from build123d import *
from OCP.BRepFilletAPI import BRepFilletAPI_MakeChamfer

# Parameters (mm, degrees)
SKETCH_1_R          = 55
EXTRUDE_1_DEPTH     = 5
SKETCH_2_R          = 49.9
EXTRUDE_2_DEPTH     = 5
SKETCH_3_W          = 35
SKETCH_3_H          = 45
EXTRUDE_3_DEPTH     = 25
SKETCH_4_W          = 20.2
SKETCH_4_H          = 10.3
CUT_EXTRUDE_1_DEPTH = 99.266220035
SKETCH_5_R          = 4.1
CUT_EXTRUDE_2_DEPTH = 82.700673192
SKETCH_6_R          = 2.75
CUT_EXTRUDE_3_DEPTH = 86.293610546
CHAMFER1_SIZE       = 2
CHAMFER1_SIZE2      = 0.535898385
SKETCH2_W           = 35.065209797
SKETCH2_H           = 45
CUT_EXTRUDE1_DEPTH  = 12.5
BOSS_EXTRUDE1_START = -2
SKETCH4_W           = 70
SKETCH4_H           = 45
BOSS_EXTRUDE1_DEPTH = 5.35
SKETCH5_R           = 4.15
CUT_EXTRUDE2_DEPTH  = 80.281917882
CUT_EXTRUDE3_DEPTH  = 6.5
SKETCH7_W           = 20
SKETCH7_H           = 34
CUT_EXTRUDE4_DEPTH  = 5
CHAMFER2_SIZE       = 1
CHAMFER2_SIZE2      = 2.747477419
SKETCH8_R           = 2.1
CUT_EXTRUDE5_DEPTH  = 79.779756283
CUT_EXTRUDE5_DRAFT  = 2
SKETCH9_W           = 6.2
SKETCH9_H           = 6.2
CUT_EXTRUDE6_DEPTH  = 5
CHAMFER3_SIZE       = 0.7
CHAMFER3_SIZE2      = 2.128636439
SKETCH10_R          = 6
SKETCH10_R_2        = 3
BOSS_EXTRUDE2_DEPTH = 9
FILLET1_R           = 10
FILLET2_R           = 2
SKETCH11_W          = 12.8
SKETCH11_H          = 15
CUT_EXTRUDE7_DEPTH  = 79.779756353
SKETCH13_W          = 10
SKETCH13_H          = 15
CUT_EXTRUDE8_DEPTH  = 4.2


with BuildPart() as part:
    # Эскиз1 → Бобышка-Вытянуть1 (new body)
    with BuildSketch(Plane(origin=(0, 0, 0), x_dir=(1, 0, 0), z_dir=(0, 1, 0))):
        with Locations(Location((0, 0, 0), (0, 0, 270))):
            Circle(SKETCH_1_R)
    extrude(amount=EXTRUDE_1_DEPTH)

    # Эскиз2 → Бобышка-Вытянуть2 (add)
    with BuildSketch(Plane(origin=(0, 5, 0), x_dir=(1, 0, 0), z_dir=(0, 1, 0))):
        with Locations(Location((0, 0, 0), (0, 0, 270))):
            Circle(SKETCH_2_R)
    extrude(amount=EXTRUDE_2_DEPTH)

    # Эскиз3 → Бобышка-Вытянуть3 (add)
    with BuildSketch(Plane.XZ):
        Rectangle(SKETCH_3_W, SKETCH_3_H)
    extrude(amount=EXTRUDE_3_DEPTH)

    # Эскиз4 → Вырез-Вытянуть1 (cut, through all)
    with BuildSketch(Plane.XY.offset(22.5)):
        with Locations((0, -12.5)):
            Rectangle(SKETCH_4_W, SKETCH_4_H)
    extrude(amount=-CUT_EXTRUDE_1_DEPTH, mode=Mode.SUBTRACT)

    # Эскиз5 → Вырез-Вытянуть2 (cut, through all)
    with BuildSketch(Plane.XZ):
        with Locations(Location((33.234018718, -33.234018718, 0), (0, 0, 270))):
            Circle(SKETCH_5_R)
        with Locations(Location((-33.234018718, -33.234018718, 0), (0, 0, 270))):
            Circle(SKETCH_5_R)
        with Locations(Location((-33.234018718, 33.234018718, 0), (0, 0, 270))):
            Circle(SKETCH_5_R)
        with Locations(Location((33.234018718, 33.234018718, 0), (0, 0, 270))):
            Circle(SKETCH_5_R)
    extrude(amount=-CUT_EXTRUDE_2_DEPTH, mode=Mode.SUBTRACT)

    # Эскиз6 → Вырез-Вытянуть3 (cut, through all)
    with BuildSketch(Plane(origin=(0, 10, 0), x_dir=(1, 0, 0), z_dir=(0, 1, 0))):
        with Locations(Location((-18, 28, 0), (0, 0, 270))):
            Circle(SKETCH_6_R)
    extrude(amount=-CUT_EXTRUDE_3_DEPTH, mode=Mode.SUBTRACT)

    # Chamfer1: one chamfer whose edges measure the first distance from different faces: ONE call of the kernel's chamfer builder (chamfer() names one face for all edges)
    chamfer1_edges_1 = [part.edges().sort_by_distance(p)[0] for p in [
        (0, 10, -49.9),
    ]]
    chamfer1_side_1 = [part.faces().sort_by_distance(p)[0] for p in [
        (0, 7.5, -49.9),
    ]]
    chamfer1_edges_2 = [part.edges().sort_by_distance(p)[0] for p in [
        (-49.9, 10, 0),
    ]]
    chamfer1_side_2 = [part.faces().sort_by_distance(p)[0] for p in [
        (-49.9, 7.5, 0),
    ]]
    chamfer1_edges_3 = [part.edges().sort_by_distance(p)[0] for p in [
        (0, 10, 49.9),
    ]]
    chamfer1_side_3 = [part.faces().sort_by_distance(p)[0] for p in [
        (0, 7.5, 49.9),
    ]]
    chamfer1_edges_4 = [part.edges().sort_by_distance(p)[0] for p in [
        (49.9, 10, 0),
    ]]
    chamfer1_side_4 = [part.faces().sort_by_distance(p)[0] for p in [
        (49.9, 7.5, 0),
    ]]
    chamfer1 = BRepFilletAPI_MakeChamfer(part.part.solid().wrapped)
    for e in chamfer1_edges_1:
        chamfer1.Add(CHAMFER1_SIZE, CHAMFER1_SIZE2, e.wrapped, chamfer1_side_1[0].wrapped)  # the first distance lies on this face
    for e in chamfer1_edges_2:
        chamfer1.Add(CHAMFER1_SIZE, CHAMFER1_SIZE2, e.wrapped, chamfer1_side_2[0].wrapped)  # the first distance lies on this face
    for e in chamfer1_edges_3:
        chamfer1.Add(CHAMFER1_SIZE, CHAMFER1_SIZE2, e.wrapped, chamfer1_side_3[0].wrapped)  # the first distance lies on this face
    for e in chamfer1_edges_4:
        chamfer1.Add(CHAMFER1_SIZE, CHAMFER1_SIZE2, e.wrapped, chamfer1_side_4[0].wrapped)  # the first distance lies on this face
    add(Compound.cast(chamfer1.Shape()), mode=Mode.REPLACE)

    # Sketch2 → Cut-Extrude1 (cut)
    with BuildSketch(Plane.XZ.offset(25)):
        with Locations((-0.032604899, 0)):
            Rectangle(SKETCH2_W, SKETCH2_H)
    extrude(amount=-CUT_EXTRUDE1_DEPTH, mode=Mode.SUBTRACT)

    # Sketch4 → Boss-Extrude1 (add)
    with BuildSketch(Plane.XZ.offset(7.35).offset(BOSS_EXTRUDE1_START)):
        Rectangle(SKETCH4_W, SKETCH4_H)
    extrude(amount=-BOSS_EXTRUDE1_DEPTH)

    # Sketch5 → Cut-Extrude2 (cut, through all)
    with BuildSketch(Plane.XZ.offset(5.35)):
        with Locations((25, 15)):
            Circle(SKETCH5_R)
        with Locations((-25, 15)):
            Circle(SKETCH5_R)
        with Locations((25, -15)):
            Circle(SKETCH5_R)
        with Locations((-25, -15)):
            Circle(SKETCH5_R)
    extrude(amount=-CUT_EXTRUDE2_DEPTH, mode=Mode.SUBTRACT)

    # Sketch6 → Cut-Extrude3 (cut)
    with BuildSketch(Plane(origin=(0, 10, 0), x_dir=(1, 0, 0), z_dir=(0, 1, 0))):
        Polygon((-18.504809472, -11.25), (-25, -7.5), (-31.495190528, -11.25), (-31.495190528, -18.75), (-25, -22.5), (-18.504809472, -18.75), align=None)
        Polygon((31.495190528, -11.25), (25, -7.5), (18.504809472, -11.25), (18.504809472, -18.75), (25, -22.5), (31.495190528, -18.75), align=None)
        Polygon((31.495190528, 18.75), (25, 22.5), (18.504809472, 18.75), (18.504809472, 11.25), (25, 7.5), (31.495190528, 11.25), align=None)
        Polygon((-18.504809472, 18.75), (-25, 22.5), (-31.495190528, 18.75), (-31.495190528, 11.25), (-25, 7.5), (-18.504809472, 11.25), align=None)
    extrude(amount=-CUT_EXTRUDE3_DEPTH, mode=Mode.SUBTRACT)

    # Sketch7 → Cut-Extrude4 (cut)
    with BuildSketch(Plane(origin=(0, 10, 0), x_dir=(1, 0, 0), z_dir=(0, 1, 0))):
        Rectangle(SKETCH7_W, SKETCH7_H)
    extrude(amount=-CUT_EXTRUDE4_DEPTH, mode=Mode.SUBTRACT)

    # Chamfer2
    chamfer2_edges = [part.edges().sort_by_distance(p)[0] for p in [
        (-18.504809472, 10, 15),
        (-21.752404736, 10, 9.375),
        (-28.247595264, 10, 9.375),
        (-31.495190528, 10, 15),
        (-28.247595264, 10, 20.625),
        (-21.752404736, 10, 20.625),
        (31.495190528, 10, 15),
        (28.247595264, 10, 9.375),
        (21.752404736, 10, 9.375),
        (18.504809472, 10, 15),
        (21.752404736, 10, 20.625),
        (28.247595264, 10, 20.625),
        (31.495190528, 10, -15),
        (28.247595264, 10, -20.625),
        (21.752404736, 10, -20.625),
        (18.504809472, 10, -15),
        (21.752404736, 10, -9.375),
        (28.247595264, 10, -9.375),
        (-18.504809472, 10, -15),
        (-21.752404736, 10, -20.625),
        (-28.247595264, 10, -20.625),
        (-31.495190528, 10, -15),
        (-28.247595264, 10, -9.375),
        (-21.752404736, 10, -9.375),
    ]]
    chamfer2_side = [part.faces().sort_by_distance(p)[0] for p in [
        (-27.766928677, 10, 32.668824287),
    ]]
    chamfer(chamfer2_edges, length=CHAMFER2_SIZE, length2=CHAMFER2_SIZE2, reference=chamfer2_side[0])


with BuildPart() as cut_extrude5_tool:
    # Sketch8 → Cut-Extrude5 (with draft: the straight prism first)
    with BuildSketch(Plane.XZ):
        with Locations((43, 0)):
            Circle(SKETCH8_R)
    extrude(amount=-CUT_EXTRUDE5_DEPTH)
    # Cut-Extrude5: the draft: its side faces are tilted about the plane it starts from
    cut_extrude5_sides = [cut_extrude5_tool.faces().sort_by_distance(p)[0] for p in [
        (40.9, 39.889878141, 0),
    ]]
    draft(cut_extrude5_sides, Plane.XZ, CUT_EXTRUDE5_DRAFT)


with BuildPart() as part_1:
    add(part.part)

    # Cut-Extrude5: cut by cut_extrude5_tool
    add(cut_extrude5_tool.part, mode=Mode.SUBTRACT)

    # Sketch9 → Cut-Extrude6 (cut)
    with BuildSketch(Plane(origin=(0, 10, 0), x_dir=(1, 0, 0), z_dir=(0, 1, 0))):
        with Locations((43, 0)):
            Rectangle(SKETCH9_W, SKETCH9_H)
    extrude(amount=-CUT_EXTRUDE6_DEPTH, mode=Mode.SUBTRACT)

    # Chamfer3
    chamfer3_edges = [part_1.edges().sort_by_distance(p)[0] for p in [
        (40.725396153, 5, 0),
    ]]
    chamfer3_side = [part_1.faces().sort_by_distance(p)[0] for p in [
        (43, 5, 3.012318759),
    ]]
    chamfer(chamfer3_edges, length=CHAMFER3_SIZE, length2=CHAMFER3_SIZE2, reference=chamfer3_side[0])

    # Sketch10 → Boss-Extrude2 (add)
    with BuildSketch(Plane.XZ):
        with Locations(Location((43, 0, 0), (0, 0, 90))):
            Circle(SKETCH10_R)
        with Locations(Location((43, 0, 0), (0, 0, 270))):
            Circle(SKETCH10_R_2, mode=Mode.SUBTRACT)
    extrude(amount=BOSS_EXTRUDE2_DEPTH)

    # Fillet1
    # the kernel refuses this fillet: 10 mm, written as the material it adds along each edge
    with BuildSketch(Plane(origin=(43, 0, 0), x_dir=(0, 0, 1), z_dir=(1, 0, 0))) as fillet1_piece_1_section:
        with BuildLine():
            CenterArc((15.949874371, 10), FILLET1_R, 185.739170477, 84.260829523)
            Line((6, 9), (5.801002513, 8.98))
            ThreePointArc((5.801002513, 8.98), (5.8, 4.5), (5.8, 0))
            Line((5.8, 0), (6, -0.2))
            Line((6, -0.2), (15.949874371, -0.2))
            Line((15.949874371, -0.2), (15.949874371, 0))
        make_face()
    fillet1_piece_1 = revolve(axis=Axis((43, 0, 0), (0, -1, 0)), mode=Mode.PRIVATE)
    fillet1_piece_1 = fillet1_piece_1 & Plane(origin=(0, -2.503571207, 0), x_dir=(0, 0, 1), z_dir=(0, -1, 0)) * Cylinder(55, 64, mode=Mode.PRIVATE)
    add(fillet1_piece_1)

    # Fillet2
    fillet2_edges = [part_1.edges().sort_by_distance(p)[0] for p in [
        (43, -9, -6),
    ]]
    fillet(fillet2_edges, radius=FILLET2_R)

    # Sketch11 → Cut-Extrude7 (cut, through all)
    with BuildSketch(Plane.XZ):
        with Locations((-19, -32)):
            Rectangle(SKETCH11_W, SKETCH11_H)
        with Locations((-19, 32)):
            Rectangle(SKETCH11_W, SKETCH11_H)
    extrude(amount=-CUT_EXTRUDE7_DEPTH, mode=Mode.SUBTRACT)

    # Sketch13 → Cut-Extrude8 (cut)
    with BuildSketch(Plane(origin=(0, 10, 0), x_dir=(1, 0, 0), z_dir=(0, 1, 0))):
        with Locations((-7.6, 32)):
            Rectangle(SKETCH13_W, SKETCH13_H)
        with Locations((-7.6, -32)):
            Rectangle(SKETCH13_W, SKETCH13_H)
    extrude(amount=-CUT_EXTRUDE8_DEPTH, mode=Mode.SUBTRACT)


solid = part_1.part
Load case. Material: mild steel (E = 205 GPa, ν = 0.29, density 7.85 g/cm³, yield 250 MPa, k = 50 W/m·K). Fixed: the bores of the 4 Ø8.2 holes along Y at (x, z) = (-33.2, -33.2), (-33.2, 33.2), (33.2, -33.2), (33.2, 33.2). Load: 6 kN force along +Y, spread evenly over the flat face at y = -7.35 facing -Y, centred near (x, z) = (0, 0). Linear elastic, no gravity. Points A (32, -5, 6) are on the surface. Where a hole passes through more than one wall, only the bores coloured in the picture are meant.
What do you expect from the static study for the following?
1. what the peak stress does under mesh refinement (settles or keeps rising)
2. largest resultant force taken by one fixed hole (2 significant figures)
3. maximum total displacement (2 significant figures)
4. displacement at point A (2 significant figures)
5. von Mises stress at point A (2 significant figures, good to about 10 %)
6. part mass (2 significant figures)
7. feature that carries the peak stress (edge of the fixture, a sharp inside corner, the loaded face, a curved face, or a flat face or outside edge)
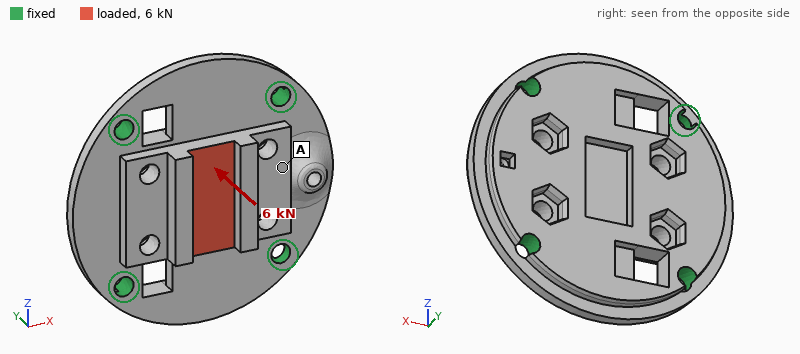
keeps rising
1.9 kN
10 µm
3.7 µm
11 MPa
740 g
edge of the fixture
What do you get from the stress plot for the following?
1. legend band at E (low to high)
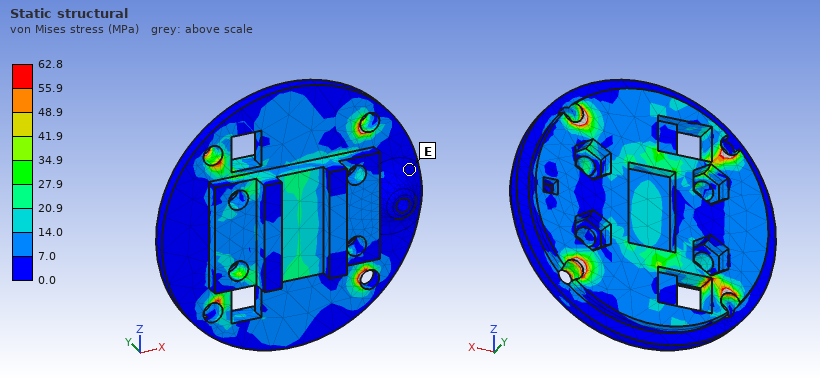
0.0 to 7.0 MPa
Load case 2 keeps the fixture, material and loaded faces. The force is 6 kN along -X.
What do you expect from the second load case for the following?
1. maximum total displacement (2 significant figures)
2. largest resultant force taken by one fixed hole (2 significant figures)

3.0 µm
2.0 kN
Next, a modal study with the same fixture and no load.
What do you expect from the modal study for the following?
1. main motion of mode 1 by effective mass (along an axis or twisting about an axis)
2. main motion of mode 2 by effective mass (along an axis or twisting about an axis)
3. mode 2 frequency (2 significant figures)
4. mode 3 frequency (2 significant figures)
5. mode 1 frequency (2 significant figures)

along Y
twisting about X
8900 Hz
9400 Hz
7500 Hz
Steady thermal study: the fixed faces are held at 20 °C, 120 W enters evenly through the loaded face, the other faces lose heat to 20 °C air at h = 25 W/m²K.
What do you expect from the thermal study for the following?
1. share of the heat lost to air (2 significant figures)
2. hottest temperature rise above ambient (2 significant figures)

16 %
79 K
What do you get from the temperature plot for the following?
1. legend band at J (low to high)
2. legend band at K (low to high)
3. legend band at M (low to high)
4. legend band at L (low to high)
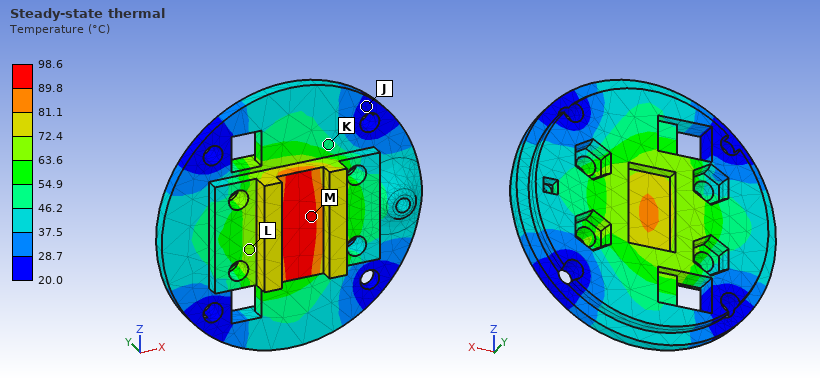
20.0 to 28.7 °C
46.2 to 54.9 °C
89.8 to 98.6 °C
63.6 to 72.4 °C
